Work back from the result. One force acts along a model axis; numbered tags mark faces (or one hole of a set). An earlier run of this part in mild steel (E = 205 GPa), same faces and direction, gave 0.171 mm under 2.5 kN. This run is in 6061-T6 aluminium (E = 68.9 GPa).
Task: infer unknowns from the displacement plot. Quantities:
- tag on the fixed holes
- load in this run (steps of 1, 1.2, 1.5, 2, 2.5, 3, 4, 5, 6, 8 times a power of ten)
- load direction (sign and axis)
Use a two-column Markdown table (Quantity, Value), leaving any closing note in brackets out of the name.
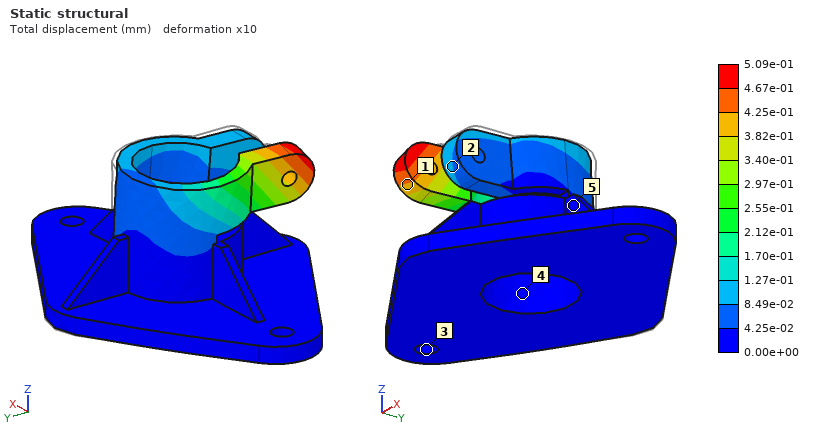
| Quantity | Value |
|---|---|
| tag on the fixed holes | 3 |
| load in this run | 2.5 kN |
| load direction | -X |
